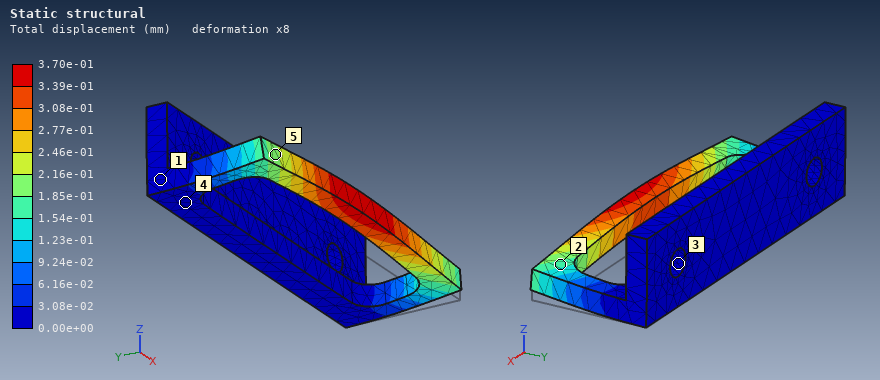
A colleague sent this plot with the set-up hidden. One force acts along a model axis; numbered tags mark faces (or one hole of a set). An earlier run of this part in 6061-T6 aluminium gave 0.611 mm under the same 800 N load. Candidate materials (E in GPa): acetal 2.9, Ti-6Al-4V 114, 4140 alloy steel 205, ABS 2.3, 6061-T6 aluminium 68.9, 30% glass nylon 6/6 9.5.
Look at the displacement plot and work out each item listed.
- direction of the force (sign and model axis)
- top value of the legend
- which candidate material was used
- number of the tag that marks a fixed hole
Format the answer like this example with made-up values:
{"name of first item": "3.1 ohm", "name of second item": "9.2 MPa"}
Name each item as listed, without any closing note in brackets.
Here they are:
{"direction of the force": "+Z", "top value of the legend": "3.70e-01 mm", "which candidate material was used": "Ti-6Al-4V", "number of the tag that marks a fixed hole": "3"}
